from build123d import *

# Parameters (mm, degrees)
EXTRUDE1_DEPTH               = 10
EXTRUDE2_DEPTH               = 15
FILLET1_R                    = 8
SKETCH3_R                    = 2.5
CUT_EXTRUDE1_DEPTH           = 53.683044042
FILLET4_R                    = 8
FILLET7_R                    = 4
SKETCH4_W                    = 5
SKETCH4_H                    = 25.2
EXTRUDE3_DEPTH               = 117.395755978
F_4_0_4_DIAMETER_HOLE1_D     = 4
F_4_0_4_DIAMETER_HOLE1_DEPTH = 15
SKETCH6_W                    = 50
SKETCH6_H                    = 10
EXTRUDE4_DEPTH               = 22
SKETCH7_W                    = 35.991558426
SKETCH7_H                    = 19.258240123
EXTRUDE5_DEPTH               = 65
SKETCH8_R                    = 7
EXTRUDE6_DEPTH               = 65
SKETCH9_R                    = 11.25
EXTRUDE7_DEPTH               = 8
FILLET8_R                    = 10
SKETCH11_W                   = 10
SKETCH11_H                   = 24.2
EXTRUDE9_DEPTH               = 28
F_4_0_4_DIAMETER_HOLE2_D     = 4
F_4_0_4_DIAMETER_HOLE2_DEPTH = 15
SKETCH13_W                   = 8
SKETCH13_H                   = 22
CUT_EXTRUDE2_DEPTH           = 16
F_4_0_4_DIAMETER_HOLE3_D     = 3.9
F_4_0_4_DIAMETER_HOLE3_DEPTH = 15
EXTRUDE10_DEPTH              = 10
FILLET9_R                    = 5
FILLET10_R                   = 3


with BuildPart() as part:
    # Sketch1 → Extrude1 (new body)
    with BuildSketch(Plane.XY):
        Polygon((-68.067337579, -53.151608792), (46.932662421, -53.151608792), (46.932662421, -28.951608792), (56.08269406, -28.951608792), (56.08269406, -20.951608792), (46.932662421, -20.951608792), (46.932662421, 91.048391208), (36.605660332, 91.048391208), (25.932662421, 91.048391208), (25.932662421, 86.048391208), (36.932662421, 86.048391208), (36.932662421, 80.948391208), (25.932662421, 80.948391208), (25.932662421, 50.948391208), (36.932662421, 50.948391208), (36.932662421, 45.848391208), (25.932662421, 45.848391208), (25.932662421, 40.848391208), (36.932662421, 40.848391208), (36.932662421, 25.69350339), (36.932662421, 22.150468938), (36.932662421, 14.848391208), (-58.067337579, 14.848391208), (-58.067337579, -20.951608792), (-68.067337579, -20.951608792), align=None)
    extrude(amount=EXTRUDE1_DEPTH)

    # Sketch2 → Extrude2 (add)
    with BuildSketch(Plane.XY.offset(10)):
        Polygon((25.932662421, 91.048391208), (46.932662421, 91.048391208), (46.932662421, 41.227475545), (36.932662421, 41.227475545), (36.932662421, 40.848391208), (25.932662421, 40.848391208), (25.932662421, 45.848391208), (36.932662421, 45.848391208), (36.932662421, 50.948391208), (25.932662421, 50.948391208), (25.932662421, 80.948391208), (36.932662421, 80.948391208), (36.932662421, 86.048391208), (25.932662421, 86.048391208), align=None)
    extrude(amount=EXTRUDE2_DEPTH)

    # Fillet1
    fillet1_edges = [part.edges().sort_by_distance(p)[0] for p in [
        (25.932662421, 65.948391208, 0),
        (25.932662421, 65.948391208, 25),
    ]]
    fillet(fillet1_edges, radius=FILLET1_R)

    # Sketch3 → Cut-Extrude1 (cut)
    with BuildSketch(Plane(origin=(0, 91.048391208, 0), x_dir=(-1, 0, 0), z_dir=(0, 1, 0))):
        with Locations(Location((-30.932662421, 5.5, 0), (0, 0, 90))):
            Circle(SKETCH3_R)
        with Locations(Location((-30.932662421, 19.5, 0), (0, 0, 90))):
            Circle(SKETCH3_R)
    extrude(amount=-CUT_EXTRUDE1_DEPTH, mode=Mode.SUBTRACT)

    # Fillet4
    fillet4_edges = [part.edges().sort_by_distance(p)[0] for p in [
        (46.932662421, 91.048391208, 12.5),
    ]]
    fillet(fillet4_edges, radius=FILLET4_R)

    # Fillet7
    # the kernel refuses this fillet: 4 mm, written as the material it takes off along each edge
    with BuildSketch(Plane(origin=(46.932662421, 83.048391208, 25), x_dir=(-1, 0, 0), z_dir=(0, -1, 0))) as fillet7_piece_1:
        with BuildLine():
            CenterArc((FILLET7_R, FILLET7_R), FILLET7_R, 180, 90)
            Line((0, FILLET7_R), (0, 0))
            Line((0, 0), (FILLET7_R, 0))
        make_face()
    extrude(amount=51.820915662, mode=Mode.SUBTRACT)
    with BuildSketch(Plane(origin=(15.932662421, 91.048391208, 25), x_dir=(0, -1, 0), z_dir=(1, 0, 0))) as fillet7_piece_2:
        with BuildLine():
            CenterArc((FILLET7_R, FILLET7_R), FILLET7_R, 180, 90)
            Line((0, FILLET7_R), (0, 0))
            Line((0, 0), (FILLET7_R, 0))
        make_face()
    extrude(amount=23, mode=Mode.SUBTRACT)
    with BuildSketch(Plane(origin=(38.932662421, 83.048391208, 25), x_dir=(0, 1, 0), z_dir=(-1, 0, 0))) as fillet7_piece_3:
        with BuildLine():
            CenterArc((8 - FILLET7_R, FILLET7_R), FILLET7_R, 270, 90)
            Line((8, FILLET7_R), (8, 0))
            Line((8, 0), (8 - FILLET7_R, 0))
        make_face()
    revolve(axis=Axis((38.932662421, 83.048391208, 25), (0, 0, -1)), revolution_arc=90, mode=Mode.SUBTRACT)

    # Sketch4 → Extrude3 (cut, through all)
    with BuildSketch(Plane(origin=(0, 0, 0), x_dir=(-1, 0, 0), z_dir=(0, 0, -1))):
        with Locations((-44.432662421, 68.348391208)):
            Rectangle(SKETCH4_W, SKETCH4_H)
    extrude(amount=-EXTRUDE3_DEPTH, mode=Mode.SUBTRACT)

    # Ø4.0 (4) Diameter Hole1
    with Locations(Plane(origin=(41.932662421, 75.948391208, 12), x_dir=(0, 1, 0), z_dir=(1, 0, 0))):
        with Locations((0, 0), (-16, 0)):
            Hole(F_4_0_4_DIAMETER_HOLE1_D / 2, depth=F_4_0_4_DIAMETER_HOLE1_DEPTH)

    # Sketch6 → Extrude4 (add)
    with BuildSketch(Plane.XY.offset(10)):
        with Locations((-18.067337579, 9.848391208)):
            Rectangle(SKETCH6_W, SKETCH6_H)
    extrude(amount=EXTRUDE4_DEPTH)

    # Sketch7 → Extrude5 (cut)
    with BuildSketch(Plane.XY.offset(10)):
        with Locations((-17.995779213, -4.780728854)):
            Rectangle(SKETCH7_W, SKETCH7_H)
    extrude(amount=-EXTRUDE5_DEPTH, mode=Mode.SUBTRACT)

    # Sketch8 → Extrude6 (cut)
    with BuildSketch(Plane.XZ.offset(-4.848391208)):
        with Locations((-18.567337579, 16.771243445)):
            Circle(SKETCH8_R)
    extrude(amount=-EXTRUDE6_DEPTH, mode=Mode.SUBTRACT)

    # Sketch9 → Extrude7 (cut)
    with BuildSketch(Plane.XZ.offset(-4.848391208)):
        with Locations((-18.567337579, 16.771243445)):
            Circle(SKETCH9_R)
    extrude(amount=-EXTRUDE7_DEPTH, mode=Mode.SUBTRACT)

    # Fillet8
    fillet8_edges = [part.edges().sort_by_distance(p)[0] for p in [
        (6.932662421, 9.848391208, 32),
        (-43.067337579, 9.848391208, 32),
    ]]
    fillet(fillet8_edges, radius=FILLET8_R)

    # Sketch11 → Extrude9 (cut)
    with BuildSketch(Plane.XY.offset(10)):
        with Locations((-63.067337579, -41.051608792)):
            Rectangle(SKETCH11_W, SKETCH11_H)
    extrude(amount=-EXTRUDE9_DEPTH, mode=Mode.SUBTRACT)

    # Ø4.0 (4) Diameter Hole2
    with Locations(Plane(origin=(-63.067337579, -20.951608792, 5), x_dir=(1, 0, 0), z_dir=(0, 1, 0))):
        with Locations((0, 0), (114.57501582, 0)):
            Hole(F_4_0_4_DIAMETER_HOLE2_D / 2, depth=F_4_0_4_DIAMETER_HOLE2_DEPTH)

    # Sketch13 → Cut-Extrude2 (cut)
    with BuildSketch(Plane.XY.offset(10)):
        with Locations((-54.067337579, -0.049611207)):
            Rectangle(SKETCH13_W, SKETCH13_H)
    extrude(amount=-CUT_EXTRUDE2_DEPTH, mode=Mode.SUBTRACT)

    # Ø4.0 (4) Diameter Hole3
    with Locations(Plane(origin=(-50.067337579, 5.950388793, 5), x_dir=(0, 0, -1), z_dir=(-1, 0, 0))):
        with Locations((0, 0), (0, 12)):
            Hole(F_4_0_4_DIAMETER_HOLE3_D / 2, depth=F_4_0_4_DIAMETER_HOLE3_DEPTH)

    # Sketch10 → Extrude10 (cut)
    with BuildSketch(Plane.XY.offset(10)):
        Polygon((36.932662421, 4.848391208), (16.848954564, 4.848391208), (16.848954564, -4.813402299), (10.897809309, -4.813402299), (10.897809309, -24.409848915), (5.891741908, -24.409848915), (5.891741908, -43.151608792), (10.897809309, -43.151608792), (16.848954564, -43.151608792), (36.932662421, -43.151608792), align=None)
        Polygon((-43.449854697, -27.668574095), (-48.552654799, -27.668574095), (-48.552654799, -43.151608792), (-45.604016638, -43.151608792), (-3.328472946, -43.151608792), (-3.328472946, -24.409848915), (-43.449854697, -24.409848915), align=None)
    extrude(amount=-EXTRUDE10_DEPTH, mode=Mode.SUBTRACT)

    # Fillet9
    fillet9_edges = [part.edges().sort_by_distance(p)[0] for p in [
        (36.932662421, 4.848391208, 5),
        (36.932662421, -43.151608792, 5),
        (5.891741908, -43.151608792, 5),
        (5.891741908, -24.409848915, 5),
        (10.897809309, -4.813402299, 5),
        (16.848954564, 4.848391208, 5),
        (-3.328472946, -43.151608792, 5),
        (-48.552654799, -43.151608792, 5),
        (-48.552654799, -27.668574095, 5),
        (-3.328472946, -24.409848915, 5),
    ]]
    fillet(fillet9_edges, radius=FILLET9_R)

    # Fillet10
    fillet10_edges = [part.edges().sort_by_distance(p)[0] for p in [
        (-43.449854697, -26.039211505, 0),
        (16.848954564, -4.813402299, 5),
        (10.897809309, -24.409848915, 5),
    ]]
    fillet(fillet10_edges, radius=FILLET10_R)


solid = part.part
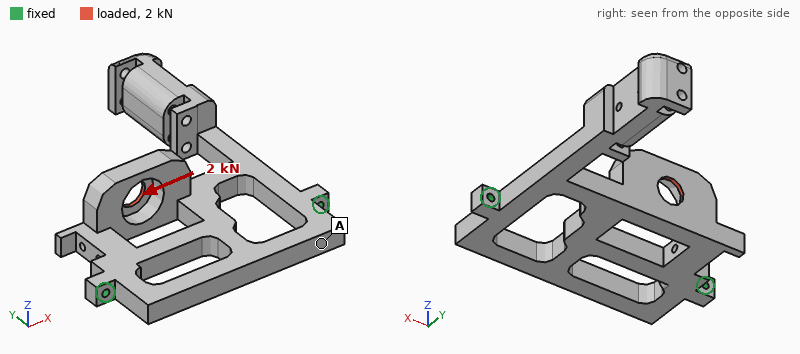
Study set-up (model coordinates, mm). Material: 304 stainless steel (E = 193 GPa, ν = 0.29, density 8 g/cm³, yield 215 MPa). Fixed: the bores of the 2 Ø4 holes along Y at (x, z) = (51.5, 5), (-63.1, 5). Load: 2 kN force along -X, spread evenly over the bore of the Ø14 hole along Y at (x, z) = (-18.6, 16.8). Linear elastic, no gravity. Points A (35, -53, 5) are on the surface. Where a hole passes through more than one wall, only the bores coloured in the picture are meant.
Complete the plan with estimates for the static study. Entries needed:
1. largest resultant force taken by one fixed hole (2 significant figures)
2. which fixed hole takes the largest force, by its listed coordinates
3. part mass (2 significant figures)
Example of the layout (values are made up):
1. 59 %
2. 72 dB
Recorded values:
1. 1.7 kN
2. (-63.1, 5)
3. 560 g
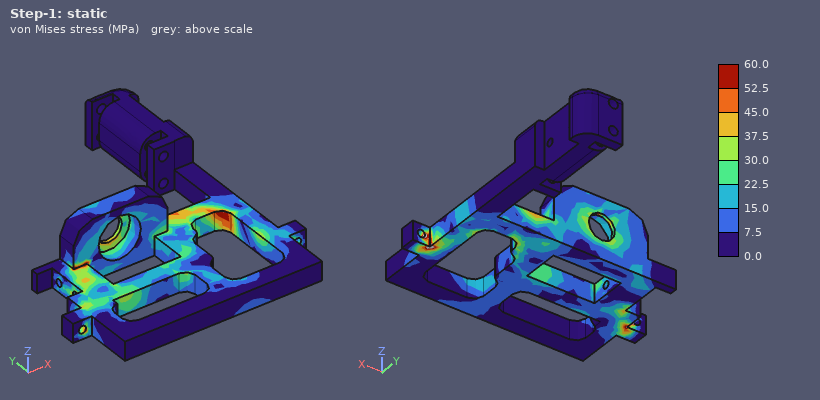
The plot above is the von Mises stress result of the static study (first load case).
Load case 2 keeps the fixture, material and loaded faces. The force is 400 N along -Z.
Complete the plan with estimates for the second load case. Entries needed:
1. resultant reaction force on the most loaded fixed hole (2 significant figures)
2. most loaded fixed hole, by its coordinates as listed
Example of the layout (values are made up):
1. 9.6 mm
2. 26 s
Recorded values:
1. 260 N
2. (-63.1, 5)
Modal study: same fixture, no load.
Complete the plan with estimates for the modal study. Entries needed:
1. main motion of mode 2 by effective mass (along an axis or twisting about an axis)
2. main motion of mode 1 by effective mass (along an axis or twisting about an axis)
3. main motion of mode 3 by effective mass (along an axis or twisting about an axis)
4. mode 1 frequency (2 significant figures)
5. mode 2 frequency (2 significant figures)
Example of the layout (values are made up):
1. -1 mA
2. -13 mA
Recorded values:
1. along X
2. along Z
3. along Z
4. 340 Hz
5. 590 Hz
